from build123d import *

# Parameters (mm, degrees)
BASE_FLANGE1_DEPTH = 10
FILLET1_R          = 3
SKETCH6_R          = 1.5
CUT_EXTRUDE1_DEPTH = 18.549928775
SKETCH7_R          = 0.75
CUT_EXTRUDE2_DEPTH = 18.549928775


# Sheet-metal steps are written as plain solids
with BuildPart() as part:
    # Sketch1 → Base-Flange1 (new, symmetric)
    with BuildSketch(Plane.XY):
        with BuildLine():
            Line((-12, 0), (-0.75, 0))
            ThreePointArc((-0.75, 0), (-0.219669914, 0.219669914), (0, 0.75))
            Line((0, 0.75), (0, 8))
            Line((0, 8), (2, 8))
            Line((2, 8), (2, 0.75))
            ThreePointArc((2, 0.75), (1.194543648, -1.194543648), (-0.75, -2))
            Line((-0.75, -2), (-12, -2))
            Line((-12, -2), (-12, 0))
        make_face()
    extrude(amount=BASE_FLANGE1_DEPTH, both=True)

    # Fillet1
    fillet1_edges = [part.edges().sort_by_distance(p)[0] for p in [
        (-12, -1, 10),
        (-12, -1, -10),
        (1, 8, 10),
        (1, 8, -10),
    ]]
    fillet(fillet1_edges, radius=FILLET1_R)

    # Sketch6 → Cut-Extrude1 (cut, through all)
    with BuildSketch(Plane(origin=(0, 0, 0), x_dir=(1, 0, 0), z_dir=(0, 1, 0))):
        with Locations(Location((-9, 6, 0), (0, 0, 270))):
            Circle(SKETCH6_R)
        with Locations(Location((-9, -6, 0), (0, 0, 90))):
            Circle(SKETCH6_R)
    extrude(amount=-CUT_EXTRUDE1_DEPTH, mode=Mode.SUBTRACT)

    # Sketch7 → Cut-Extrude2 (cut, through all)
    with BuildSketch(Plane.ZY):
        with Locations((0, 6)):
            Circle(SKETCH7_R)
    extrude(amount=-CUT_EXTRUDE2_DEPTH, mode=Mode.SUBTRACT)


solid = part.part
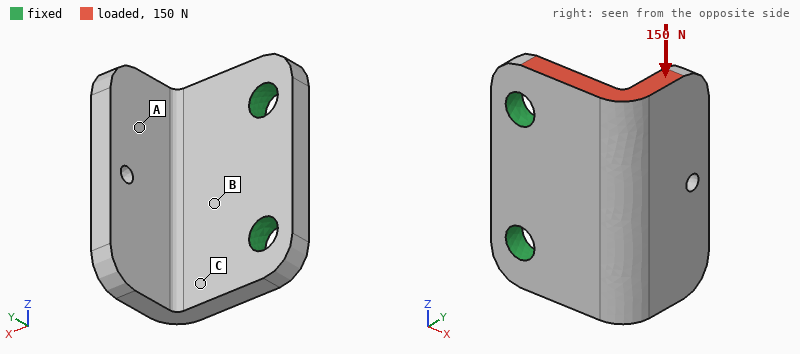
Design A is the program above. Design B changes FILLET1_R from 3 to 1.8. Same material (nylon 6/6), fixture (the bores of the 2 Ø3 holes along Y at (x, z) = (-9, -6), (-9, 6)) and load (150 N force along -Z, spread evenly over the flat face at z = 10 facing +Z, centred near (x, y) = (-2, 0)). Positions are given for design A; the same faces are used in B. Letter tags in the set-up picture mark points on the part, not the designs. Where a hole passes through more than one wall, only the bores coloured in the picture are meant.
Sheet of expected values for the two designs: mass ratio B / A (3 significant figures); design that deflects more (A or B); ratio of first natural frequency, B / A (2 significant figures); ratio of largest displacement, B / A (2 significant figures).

1.01
B
0.99
1.3
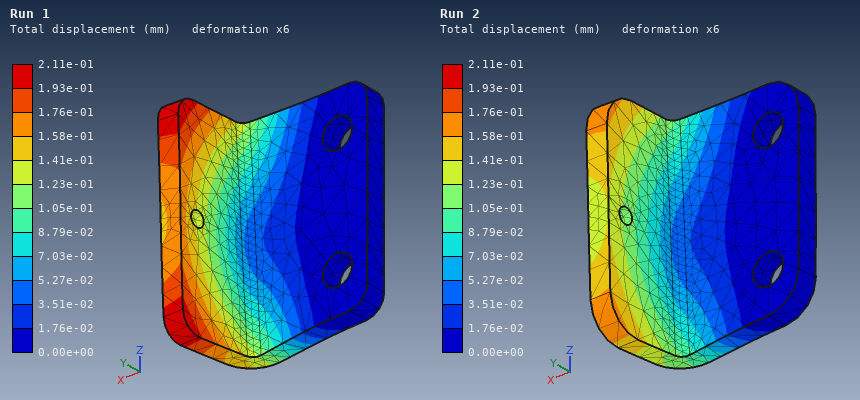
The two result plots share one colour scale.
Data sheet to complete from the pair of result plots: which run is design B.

Run 1
